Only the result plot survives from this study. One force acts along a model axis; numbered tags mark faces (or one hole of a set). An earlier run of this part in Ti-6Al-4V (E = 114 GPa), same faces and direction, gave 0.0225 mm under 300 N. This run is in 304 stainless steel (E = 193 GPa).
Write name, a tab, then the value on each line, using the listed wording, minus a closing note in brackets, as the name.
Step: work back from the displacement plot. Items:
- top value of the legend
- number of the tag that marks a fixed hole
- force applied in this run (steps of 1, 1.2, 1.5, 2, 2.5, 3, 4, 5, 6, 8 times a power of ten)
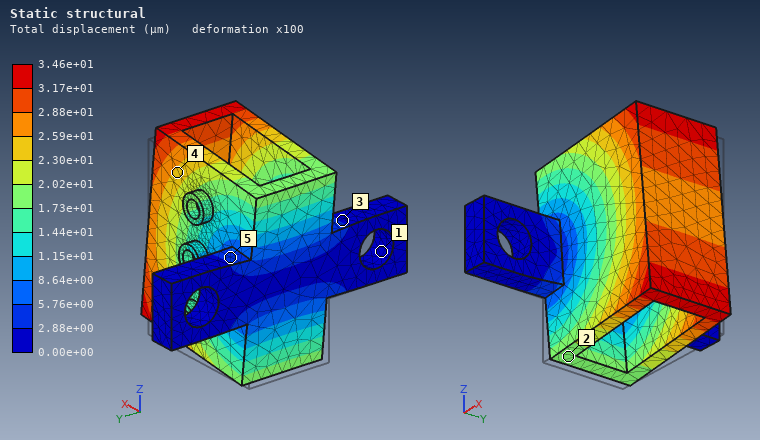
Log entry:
top value of the legend	3.46e+01 µm
number of the tag that marks a fixed hole	1
force applied in this run	800 N
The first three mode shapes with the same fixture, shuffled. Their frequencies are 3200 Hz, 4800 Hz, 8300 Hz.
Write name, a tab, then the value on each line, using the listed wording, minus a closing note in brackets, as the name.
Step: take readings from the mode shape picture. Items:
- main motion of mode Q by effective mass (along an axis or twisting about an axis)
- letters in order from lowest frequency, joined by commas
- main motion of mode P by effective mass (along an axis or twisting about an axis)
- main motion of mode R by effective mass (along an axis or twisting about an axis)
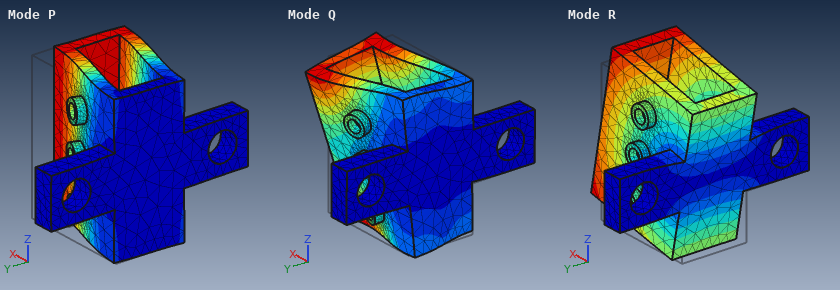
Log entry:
main motion of mode Q by effective mass	twisting about X
letters in order from lowest frequency, joined by commas	R, P, Q
main motion of mode P by effective mass	along Y
main motion of mode R by effective mass	along Z
